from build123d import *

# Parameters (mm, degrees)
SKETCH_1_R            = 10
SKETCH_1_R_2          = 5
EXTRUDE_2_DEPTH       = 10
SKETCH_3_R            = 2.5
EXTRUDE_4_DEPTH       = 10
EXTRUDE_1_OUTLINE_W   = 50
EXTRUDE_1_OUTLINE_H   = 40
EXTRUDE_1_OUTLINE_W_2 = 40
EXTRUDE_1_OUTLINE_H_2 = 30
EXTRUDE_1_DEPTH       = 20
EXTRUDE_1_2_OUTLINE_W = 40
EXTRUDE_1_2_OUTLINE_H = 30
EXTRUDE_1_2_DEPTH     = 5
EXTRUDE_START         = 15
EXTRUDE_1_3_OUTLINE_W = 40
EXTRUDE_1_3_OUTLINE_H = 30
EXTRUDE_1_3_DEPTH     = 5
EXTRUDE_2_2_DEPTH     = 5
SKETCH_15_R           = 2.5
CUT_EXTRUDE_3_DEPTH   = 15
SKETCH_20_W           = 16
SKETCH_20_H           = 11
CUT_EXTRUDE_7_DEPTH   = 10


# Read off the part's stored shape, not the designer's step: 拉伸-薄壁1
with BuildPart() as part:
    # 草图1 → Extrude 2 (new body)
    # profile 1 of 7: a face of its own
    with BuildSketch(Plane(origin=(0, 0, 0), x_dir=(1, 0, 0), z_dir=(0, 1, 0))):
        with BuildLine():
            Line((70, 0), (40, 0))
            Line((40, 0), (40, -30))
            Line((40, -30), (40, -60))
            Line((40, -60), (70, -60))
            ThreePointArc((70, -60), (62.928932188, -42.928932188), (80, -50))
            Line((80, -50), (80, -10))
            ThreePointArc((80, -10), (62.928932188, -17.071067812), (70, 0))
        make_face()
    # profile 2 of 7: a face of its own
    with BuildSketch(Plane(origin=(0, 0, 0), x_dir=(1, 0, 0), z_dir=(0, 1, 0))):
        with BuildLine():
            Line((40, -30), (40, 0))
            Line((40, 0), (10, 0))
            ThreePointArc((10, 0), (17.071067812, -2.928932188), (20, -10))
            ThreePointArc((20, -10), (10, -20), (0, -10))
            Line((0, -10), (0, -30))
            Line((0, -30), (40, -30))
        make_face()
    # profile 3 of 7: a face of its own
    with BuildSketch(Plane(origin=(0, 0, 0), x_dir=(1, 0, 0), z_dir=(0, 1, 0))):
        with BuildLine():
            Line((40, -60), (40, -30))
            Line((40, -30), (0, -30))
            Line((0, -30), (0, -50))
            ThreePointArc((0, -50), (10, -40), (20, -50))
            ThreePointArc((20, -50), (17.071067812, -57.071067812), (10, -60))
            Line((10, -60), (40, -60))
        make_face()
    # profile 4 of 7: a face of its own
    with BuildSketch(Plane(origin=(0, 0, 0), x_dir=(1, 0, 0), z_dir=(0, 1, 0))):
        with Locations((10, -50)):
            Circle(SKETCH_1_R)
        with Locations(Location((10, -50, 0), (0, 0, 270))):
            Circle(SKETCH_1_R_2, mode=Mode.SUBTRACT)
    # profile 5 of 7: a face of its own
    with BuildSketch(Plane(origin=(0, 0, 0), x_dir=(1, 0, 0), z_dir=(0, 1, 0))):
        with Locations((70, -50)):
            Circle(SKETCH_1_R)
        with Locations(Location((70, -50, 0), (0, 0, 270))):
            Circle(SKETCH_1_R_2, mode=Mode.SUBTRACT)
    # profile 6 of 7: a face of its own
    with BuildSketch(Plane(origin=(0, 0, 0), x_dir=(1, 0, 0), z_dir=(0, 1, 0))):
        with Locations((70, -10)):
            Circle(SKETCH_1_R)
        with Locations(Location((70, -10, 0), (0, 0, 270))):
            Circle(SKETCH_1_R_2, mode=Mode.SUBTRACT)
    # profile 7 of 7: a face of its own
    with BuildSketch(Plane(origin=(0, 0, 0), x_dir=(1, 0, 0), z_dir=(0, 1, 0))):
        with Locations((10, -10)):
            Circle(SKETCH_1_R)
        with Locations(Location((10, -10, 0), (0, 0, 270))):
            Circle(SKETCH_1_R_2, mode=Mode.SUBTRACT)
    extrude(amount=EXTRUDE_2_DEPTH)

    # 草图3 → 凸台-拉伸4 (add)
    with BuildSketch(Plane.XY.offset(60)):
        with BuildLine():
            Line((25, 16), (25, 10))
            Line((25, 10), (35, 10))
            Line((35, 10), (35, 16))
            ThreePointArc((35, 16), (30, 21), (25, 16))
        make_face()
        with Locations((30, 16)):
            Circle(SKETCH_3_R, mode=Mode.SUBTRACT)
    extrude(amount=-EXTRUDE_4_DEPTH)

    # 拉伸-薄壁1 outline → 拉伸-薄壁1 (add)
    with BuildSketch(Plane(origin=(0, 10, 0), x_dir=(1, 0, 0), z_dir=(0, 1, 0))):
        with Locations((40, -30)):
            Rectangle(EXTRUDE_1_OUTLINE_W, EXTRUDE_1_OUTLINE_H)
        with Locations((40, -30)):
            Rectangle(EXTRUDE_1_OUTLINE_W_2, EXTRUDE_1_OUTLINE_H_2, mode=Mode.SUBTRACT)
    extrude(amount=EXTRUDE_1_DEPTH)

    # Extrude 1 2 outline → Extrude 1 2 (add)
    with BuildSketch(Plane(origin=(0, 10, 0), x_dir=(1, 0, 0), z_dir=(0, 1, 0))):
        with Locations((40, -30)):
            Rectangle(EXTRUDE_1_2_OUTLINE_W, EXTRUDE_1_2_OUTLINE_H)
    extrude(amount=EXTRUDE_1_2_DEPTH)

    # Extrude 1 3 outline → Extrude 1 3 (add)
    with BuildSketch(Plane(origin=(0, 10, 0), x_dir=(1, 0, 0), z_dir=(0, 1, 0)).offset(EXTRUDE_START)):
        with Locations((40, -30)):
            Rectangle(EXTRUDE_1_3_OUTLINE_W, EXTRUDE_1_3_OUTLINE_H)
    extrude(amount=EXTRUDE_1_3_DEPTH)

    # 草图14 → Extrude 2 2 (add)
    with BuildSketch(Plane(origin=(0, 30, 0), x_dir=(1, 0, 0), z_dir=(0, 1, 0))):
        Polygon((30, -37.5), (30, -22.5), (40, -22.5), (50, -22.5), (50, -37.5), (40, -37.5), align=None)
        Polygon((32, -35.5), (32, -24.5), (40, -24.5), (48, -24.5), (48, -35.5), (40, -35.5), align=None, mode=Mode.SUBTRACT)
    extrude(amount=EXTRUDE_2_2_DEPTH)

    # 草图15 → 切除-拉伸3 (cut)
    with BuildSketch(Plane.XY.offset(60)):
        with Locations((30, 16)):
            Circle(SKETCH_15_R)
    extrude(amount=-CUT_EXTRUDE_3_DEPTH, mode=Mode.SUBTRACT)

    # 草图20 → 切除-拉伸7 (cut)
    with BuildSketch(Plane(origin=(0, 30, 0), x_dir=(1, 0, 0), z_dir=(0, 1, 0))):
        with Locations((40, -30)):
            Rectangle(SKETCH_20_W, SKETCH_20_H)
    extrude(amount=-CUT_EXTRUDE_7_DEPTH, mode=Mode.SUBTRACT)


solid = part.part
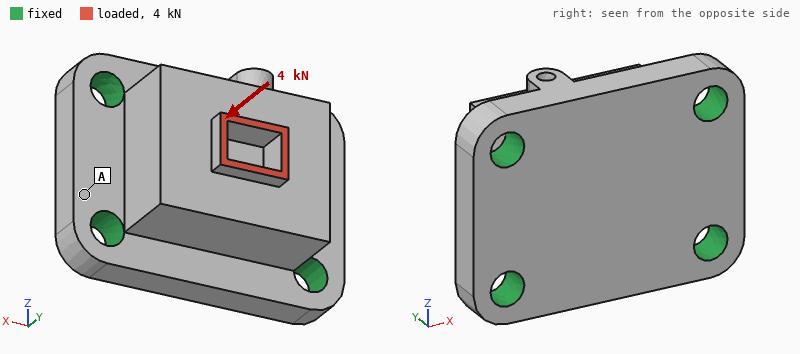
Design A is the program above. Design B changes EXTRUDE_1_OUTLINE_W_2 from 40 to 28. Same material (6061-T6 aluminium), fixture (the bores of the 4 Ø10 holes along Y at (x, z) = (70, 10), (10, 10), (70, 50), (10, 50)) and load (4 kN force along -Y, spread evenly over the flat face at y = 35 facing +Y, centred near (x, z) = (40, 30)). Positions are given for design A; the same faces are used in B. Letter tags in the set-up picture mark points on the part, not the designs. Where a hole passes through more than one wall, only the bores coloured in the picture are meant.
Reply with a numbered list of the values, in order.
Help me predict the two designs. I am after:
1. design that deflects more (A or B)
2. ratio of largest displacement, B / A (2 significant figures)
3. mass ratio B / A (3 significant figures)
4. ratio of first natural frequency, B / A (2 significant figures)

1. A
2. 0.65
3. 1.05
4. 1.0
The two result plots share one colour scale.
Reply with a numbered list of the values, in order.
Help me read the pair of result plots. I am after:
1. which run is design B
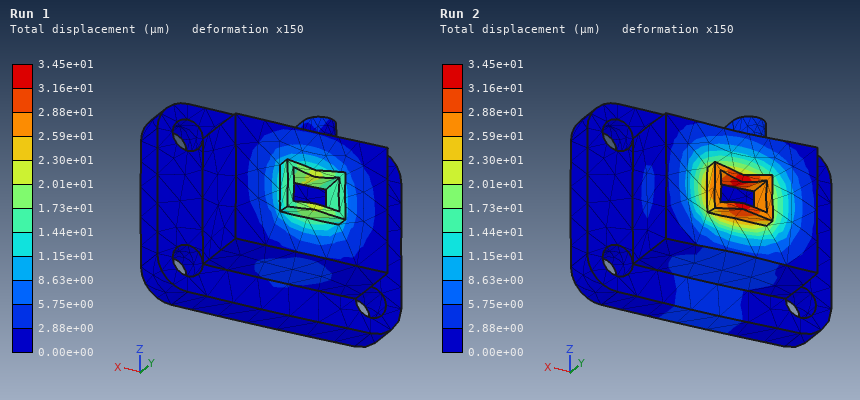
1. Run 1
